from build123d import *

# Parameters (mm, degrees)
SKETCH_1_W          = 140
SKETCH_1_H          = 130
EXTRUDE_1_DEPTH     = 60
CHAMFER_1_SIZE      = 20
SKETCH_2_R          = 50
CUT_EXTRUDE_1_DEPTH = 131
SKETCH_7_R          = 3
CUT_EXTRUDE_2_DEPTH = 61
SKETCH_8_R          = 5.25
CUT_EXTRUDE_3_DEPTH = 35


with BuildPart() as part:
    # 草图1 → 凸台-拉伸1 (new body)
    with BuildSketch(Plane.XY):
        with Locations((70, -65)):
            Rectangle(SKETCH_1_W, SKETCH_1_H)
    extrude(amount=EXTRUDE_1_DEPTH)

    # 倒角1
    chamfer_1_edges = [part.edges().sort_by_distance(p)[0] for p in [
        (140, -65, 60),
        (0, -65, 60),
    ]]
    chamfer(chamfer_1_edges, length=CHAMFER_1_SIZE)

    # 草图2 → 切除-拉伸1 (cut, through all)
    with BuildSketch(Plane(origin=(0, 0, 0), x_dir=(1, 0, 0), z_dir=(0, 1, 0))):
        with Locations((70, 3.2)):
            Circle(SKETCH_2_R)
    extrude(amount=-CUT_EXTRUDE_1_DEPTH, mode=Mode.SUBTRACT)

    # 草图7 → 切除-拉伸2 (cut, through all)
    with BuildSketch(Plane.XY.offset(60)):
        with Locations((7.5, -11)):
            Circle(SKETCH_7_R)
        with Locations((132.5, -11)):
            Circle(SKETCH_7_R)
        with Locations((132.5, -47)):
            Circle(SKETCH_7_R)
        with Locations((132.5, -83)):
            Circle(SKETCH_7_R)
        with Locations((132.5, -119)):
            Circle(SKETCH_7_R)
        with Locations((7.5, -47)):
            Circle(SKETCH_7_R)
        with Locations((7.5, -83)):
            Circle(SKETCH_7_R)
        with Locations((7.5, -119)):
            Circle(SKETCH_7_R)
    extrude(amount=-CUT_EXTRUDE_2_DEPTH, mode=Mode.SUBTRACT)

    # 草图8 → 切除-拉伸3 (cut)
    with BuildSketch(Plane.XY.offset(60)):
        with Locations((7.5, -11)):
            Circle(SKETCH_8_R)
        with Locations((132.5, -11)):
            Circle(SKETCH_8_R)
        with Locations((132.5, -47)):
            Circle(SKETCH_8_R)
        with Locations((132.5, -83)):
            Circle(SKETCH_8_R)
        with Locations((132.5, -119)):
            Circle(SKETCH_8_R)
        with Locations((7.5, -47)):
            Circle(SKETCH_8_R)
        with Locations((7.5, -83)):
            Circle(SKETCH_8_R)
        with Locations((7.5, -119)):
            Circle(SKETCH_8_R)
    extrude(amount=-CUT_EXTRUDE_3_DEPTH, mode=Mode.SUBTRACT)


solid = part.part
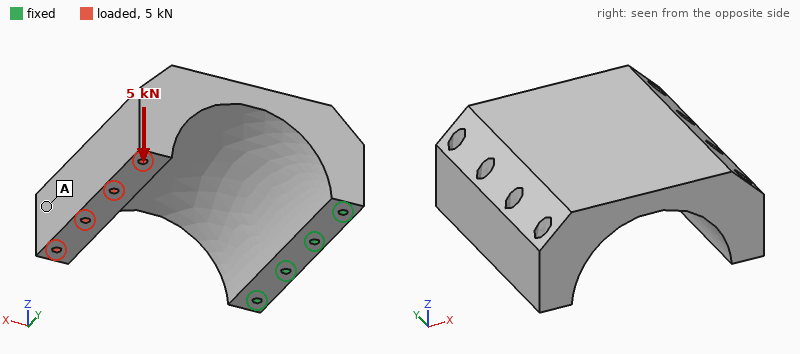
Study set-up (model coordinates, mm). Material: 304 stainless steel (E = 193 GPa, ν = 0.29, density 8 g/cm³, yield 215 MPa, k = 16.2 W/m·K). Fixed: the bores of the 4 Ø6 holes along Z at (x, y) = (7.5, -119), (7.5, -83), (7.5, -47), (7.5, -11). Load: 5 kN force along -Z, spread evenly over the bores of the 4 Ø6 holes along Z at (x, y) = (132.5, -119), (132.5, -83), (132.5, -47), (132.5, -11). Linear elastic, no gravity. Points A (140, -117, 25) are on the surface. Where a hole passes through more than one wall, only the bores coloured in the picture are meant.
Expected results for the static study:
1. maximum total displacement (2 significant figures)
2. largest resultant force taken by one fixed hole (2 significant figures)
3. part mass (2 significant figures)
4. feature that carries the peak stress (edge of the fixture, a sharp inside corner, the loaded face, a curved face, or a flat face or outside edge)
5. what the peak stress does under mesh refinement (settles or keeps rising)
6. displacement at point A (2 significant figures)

0.33 mm
2.1 kN
4.4 kg
edge of the fixture
keeps rising
0.30 mm
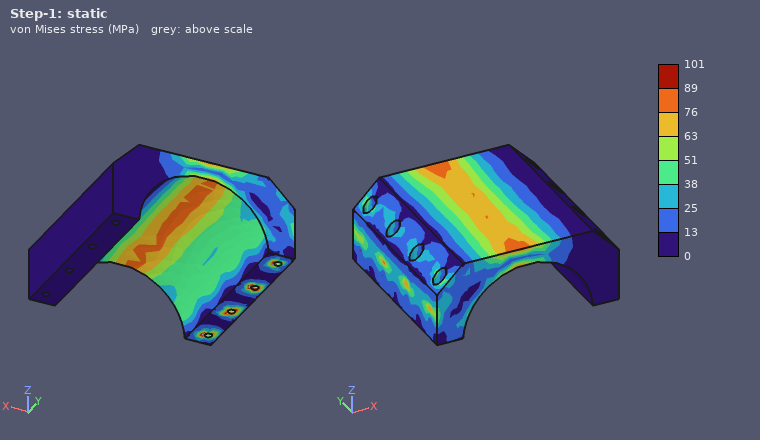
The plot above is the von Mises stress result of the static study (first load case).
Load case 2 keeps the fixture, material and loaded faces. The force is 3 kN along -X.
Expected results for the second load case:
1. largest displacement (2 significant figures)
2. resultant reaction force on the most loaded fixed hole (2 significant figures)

94 µm
810 N
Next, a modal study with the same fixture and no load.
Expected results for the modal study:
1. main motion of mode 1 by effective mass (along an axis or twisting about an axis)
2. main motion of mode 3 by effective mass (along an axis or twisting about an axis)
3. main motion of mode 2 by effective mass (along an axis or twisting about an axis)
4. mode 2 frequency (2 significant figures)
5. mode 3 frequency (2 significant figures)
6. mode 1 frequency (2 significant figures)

along Z
along X
along Y
1200 Hz
1900 Hz
560 Hz
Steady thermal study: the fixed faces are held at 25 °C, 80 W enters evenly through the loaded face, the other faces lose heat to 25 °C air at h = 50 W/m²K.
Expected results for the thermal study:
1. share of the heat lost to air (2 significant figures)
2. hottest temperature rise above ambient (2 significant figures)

94 %
76 K
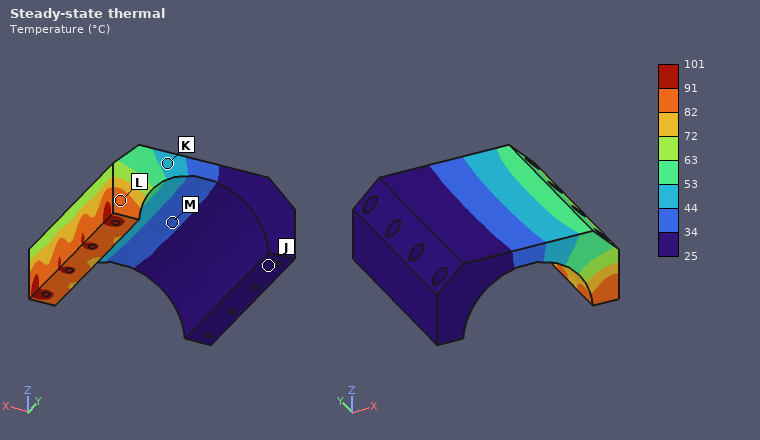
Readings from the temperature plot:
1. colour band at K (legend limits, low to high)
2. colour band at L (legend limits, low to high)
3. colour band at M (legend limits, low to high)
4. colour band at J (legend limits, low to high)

44 to 53 °C
82 to 91 °C
34 to 44 °C
25 to 34 °C
